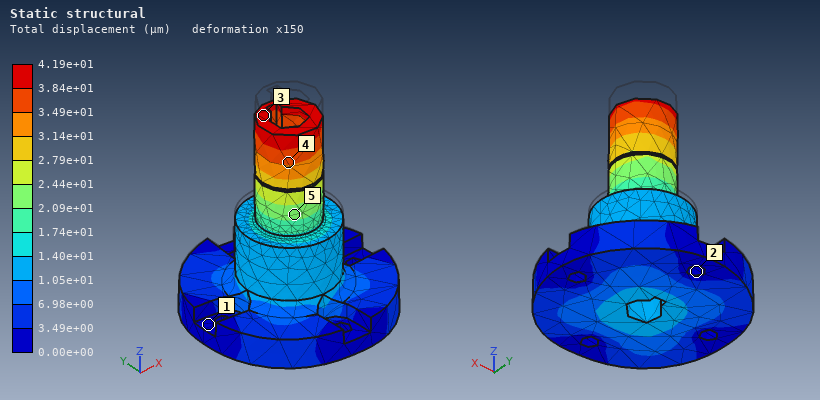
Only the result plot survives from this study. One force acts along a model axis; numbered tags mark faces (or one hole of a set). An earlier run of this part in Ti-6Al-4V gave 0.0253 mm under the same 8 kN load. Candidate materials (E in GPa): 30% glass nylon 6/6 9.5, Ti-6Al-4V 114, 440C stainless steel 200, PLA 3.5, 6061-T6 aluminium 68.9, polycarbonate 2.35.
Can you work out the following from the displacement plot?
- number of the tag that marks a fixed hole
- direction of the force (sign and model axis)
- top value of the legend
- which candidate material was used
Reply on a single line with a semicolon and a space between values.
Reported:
2; -Z; 4.19e+01 µm; 6061-T6 aluminium
